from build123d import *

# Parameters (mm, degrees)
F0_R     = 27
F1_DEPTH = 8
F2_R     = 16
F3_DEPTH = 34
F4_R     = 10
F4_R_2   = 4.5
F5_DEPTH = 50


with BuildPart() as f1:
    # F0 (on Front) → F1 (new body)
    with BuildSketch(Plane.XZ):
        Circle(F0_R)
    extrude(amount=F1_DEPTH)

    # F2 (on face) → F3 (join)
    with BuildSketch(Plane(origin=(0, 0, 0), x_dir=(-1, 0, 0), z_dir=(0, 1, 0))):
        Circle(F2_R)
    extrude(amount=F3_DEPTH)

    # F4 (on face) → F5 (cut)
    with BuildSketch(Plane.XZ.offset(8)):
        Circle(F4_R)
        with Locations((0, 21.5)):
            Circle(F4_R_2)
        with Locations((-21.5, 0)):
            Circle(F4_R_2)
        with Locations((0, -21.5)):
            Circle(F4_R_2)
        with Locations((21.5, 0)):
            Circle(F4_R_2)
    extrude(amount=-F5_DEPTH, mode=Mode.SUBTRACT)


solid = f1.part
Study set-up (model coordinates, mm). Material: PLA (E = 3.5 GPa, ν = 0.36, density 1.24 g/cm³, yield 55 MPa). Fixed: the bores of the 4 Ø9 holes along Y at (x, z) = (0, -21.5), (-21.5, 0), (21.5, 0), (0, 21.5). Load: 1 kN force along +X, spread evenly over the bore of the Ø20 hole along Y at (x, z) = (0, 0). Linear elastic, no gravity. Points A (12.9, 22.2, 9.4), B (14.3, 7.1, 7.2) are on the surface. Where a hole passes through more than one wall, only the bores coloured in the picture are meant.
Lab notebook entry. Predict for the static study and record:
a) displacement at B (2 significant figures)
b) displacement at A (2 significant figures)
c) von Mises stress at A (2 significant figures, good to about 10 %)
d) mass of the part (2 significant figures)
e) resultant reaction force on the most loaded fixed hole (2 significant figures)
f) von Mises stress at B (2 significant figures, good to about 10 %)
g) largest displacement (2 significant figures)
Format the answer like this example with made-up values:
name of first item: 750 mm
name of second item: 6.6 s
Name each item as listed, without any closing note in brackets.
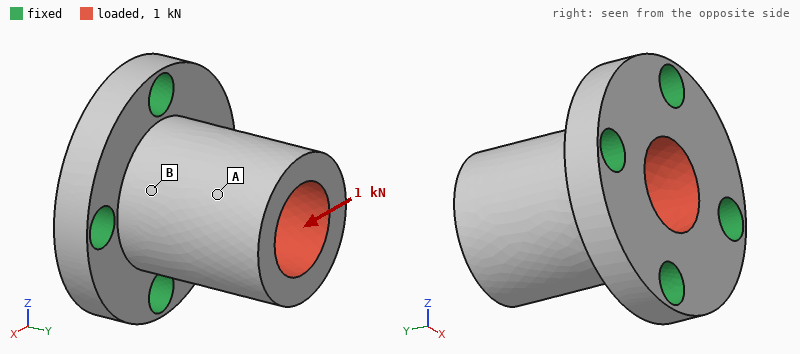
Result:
displacement at B: 0.036 mm
displacement at A: 0.076 mm
von Mises stress at A: 1.2 MPa
mass of the part: 38 g
resultant reaction force on the most loaded fixed hole: 530 N
von Mises stress at B: 3.1 MPa
largest displacement: 0.11 mm
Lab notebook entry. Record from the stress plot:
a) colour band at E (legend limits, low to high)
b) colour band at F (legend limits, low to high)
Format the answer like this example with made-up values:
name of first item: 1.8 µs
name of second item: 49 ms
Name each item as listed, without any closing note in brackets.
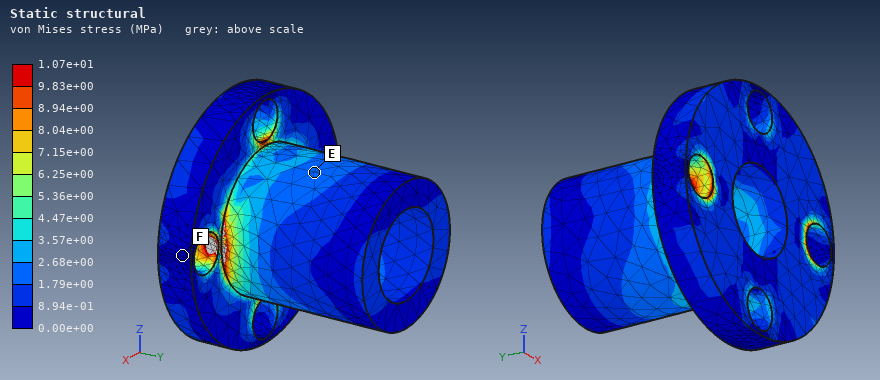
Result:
colour band at E: 1.79e+00 to 2.68e+00 MPa
colour band at F: 0.00e+00 to 8.94e-01 MPa
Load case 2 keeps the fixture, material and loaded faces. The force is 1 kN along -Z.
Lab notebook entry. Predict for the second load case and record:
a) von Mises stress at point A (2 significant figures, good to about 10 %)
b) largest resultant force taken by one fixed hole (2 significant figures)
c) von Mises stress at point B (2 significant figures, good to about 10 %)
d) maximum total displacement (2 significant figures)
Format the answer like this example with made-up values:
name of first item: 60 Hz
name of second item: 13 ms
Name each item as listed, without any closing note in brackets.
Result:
von Mises stress at point A: 1.5 MPa
largest resultant force taken by one fixed hole: 540 N
von Mises stress at point B: 2.7 MPa
maximum total displacement: 0.11 mm
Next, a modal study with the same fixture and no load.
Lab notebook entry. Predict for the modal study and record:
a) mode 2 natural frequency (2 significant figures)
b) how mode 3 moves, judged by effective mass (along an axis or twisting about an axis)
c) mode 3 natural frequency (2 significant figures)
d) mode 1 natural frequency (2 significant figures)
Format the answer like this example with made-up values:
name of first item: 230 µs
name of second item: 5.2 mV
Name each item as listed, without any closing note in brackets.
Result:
mode 2 natural frequency: 3600 Hz
how mode 3 moves, judged by effective mass: twisting about Y
mode 3 natural frequency: 6800 Hz
mode 1 natural frequency: 3600 Hz
